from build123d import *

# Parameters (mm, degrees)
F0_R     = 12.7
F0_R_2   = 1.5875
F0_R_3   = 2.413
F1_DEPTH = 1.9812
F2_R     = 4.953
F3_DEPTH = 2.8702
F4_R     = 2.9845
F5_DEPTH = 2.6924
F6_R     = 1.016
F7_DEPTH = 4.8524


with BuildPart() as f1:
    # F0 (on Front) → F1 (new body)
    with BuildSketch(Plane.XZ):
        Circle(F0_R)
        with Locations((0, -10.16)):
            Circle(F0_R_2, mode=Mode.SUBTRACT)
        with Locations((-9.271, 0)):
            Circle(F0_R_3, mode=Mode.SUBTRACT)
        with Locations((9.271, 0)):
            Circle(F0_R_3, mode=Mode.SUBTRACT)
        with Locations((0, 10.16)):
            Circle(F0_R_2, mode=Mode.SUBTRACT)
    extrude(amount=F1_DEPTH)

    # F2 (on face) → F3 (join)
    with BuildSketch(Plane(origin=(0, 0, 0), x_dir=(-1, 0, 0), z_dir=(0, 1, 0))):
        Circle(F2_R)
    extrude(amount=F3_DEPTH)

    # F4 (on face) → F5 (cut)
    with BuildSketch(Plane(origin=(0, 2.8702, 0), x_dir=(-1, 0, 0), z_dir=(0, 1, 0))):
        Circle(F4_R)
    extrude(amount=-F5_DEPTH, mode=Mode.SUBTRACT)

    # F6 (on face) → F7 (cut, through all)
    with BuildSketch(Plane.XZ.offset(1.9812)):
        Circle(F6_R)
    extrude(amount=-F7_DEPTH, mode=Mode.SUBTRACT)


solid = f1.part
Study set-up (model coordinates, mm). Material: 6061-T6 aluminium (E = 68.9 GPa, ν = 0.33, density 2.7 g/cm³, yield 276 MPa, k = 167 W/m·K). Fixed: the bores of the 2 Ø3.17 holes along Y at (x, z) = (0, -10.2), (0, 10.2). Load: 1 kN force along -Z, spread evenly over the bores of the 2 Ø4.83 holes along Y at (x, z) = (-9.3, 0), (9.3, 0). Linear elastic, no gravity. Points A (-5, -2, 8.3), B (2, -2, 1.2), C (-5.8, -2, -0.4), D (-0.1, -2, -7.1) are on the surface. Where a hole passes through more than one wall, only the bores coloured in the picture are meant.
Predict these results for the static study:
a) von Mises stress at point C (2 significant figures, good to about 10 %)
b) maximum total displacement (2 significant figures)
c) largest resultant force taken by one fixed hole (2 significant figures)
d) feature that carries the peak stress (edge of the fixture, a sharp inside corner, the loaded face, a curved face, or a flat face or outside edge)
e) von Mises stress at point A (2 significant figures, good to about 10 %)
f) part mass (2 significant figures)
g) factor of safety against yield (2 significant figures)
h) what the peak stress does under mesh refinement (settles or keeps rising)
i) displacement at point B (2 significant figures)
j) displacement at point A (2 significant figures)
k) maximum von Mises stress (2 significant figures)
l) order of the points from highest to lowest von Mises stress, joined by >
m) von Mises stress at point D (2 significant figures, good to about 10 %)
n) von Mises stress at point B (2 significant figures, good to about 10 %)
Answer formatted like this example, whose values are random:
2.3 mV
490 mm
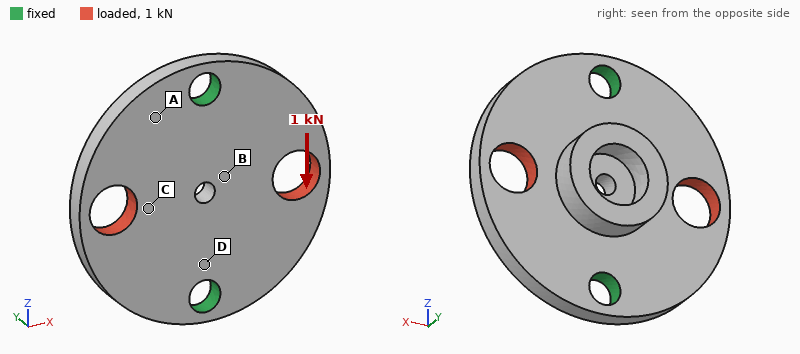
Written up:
38 MPa
9.2 µm
500 N
the loaded face
20 MPa
2.8 g
3.8
settles
2.3 µm
2.6 µm
72 MPa
C > D > A > B
28 MPa
13 MPa
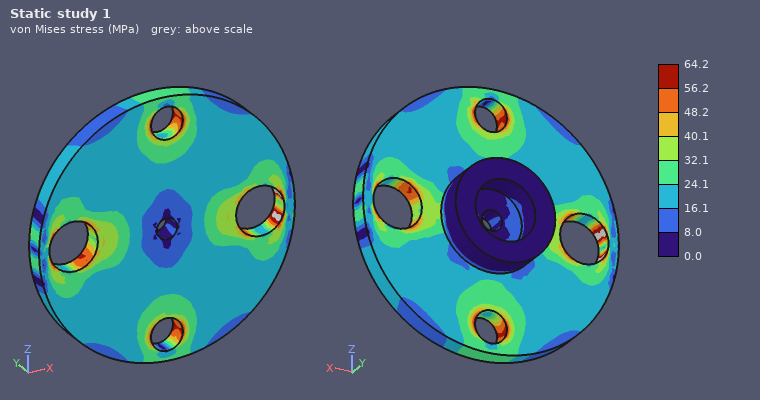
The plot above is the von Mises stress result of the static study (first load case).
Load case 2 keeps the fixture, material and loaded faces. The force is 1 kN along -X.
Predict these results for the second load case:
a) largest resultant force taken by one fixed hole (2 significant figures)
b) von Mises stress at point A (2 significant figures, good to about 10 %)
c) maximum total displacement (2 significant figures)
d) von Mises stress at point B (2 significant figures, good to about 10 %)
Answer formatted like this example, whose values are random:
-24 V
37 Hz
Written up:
500 N
22 MPa
8.7 µm
10 MPa
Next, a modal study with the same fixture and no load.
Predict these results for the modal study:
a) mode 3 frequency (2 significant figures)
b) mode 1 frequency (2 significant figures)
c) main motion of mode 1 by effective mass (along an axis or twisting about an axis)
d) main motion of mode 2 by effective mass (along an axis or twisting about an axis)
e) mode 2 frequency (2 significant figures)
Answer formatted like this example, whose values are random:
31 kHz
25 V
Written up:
28 kHz
11 kHz
twisting about Z
along Y
16 kHz
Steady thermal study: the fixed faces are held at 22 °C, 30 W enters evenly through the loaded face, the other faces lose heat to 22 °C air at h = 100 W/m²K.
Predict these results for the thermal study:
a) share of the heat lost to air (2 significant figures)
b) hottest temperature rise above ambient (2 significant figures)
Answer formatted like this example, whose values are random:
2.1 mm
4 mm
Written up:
6.9 %
42 K
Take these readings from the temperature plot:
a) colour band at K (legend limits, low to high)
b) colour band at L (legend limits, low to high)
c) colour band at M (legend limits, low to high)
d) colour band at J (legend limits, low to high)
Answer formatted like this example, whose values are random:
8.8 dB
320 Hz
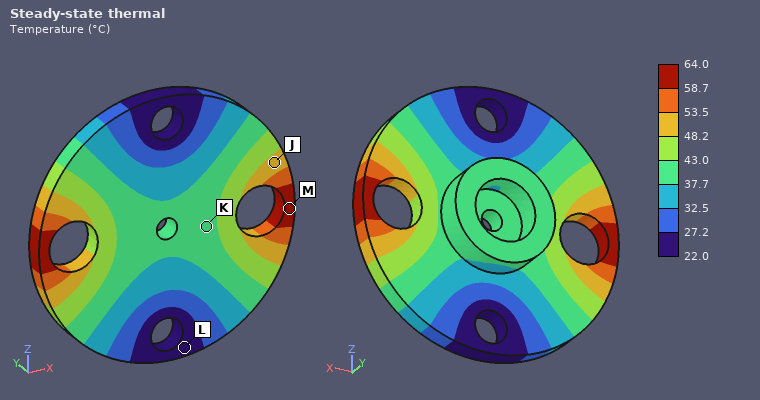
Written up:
37.7 to 43.0 °C
22.0 to 27.2 °C
58.7 to 64.0 °C
48.2 to 53.5 °C
